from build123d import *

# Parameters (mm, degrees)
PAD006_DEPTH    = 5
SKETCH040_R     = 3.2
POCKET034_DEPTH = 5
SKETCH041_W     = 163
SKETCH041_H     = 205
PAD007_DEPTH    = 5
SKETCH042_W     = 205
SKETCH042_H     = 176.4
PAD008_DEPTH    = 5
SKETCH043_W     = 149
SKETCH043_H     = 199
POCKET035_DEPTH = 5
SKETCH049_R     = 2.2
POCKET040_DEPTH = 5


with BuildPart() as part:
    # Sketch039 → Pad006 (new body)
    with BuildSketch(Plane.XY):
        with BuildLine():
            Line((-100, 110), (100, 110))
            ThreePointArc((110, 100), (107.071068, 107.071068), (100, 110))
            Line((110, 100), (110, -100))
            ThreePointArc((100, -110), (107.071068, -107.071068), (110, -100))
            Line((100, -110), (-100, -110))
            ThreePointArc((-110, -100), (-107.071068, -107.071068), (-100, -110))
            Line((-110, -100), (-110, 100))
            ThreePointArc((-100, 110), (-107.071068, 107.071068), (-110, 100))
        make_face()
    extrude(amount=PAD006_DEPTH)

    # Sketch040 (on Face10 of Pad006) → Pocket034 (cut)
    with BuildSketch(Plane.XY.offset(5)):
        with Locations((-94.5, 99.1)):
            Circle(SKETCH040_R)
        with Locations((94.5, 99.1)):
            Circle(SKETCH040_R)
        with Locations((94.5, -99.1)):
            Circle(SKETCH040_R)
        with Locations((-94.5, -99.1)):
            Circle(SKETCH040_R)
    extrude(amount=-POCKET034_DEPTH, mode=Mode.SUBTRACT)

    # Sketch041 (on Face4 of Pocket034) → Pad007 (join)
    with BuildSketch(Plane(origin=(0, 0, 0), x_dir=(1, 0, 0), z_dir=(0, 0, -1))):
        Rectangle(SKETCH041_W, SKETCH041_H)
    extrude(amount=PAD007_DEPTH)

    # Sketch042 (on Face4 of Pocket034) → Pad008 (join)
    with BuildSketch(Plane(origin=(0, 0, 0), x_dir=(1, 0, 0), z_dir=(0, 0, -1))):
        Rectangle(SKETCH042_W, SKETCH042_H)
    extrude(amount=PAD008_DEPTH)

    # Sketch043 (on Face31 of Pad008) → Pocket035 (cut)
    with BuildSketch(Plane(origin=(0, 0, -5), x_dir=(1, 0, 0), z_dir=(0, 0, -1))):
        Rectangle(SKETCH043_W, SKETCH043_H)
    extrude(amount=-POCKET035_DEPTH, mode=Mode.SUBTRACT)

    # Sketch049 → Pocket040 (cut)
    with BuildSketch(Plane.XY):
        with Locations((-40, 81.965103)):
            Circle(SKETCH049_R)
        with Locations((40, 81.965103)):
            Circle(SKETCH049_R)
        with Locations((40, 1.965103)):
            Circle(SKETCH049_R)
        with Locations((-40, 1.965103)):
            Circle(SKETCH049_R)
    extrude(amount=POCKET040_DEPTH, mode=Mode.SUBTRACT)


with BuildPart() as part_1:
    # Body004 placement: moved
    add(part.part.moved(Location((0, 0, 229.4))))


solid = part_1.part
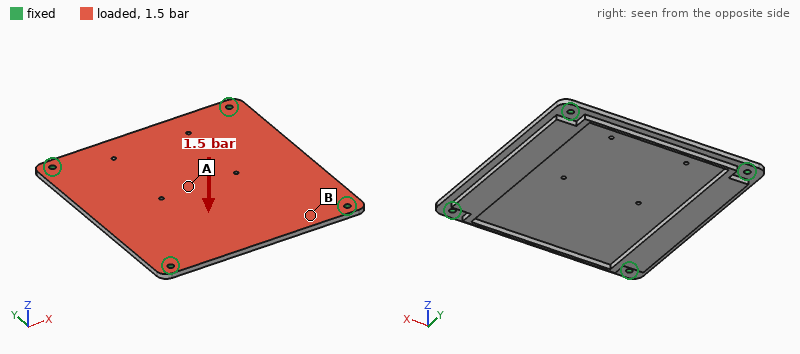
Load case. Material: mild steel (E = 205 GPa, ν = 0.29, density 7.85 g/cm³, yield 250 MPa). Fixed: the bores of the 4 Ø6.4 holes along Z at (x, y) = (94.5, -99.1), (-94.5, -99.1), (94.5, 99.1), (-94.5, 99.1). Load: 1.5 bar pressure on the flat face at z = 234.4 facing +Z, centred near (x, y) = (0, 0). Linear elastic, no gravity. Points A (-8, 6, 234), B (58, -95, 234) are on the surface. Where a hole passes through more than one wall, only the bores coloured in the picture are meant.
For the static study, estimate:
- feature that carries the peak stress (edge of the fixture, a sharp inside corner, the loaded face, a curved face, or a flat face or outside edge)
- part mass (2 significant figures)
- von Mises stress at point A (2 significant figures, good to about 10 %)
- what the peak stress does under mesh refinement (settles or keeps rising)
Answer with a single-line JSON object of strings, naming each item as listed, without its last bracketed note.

{"feature that carries the peak stress": "edge of the fixture", "part mass": "2.3 kg", "von Mises stress at point A": "61 MPa", "what the peak stress does under mesh refinement": "keeps rising"}
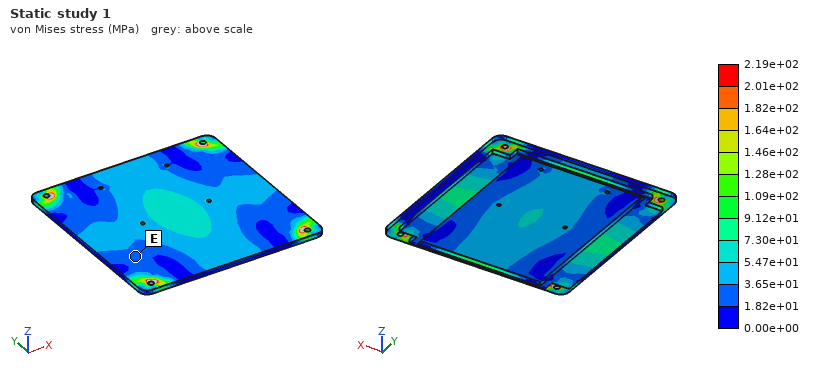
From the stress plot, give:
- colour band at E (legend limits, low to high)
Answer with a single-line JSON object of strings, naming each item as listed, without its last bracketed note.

{"colour band at E": "1.82e+01 to 3.65e+01 MPa"}
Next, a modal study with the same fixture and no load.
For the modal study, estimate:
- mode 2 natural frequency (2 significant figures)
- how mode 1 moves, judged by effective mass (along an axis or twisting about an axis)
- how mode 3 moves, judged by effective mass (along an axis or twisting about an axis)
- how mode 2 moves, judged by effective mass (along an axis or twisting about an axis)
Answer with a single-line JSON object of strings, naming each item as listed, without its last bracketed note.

{"mode 2 natural frequency": "930 Hz", "how mode 1 moves, judged by effective mass": "along Z", "how mode 3 moves, judged by effective mass": "twisting about X", "how mode 2 moves, judged by effective mass": "twisting about Y"}
